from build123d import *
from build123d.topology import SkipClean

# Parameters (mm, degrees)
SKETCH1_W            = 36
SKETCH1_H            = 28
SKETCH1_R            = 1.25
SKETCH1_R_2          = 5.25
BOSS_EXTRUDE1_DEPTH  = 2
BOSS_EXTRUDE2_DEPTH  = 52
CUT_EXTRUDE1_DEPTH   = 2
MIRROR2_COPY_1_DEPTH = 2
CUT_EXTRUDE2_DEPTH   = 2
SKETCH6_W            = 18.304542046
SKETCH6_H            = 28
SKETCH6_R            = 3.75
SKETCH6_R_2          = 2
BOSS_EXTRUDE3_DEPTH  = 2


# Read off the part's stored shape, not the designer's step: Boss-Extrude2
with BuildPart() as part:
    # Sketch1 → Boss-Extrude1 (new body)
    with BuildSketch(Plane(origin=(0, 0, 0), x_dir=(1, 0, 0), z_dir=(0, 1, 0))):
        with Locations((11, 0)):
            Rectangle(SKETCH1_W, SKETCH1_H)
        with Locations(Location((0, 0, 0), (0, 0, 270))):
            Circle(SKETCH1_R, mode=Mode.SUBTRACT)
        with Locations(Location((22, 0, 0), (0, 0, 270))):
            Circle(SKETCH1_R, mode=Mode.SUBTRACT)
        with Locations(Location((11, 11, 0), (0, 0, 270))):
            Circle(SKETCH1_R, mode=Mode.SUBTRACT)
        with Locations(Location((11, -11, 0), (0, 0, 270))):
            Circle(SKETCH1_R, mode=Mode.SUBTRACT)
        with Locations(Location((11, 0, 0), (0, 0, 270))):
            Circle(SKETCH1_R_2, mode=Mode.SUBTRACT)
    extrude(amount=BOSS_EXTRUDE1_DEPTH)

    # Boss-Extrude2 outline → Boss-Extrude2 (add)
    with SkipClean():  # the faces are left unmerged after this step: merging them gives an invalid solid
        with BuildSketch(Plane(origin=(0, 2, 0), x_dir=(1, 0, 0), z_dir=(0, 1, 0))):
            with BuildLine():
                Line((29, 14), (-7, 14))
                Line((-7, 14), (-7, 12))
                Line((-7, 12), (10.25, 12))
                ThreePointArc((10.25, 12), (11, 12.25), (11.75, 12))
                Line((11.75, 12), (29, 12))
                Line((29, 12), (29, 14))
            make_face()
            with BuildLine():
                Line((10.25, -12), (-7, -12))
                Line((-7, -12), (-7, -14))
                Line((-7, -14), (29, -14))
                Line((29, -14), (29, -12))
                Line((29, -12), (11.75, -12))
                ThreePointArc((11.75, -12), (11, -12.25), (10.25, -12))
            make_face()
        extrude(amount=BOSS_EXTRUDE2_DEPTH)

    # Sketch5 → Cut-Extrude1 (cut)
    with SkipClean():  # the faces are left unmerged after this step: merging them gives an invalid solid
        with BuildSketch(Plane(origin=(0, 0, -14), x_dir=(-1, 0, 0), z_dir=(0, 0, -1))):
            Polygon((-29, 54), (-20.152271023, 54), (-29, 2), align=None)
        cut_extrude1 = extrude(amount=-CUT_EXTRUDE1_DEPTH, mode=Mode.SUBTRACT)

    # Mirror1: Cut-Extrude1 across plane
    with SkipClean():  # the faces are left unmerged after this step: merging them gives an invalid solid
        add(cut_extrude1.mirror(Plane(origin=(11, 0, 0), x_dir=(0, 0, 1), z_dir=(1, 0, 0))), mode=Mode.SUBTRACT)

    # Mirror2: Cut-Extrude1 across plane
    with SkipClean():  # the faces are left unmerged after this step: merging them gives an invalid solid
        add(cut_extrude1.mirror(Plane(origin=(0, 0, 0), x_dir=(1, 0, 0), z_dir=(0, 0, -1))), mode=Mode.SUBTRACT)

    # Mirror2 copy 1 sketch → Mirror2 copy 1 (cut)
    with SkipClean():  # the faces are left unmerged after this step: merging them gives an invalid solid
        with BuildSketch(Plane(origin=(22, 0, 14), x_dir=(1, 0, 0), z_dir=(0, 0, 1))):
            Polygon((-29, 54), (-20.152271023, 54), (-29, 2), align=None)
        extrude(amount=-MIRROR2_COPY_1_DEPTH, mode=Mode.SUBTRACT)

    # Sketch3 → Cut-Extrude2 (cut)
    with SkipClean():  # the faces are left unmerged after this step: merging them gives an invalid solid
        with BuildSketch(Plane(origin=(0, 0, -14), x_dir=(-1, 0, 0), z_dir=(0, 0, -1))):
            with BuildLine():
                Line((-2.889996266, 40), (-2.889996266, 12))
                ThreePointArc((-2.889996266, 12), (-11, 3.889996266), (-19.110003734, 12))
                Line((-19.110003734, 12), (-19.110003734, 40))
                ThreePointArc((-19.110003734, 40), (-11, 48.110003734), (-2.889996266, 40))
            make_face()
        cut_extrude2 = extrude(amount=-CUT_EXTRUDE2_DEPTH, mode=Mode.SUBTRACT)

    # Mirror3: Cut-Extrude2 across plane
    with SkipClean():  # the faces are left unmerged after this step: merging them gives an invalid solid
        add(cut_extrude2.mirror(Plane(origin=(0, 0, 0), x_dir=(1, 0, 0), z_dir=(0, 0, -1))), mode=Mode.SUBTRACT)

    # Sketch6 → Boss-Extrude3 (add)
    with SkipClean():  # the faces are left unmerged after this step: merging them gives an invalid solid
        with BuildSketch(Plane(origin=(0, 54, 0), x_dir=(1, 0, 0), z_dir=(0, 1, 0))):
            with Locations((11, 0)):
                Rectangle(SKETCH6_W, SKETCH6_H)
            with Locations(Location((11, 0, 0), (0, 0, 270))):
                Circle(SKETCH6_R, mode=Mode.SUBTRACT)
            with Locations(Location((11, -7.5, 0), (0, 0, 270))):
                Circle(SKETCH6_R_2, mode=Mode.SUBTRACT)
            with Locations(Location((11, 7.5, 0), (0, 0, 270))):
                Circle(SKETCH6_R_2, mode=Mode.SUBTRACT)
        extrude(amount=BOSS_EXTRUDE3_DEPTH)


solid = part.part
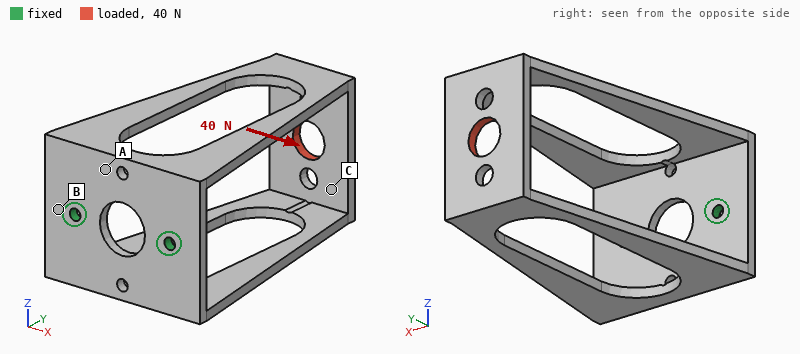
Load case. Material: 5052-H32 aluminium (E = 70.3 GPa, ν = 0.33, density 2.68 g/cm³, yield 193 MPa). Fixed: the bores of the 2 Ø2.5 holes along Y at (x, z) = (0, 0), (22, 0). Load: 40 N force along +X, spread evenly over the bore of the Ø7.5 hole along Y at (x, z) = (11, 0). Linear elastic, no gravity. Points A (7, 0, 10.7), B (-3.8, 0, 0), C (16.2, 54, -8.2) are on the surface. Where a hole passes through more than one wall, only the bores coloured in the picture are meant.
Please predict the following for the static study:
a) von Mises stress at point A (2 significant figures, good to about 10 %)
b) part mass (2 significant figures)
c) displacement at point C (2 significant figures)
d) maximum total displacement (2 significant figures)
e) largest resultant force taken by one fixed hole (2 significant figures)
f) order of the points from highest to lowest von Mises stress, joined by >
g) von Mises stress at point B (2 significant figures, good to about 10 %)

15 MPa
15 g
0.11 mm
0.12 mm
82 N
B > A > C
32 MPa
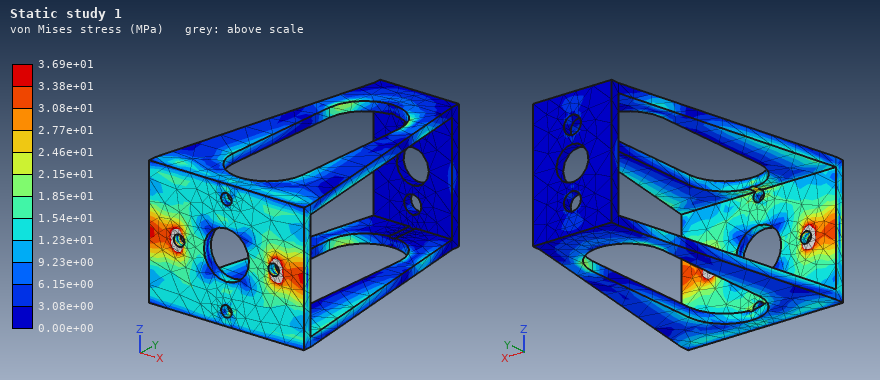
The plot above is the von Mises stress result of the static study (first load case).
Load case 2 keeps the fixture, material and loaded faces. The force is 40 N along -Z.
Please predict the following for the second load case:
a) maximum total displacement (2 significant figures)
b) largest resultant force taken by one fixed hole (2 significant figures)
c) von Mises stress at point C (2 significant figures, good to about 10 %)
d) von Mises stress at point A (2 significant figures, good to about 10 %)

0.77 mm
20 N
28 MPa
23 MPa
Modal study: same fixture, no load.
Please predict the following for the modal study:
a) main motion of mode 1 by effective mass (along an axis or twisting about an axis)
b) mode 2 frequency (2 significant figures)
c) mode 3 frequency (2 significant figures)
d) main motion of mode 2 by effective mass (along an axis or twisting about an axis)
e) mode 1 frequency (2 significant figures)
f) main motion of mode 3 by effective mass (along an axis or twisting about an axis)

along Z
1300 Hz
1800 Hz
along X
520 Hz
twisting about Y
